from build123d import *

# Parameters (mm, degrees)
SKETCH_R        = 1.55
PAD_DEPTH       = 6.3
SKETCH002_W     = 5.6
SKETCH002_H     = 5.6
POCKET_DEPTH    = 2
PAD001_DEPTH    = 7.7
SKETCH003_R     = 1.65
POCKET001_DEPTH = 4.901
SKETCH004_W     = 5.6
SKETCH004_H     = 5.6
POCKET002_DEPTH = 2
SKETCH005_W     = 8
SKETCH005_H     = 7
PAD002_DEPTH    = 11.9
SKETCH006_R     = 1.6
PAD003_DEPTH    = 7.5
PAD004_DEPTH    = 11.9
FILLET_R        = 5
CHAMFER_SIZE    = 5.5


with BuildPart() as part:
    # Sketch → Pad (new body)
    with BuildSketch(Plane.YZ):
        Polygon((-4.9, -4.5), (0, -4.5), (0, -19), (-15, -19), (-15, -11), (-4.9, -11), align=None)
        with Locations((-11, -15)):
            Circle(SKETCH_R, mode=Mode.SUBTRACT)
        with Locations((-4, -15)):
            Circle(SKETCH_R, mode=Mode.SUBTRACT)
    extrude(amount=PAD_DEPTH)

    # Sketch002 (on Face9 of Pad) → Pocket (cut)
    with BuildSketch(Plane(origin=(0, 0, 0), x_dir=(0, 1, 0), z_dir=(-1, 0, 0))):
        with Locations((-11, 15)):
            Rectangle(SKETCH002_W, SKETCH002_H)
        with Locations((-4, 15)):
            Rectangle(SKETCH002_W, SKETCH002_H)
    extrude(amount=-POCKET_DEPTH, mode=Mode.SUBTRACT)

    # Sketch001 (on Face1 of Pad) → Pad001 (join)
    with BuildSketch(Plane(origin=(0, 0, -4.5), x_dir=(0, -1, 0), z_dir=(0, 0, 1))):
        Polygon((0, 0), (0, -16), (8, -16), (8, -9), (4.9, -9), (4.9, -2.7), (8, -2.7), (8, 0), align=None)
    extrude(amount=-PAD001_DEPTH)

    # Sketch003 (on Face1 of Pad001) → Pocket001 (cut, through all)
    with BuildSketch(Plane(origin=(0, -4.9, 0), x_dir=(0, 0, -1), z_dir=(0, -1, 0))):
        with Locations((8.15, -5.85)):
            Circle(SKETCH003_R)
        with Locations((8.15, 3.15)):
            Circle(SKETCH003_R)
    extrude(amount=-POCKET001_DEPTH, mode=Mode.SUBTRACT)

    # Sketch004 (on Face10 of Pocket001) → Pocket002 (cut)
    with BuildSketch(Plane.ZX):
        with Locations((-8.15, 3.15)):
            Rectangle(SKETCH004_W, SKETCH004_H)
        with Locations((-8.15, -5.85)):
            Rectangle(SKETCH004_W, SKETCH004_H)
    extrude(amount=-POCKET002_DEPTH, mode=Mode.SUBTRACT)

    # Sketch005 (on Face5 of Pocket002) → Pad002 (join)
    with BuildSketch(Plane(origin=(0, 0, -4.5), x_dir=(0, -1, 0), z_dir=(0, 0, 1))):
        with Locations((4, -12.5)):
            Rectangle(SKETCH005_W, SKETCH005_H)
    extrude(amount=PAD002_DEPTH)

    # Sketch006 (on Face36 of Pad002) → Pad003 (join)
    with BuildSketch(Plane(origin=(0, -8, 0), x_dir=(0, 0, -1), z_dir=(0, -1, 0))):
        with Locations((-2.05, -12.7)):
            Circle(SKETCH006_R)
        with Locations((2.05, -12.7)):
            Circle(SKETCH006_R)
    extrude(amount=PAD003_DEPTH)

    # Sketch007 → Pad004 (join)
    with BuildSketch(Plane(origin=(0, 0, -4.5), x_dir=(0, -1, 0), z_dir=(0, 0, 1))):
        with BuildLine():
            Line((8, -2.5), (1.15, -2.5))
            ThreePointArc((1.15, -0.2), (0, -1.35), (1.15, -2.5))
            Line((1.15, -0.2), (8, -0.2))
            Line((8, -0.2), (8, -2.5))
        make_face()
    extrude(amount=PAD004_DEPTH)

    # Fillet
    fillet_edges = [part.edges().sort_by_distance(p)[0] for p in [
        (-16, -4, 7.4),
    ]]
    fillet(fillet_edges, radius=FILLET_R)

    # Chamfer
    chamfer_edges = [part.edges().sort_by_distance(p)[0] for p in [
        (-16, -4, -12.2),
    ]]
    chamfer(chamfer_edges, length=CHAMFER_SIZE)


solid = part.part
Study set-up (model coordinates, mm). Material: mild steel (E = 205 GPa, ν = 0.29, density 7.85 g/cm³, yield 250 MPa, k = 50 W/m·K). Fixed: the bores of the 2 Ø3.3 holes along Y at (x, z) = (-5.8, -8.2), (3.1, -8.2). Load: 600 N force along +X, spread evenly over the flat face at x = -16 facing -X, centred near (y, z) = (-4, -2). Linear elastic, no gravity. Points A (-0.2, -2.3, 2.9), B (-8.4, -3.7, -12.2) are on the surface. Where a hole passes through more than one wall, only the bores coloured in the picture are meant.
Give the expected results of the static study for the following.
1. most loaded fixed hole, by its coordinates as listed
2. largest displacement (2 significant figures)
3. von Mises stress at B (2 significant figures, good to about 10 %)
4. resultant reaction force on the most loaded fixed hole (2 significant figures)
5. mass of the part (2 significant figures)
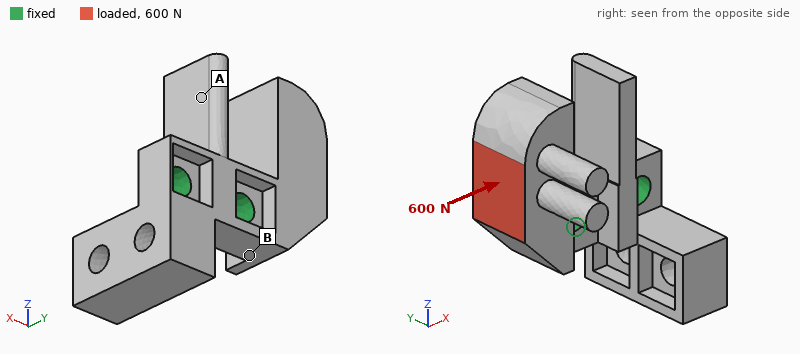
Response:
(-5.8, -8.2)
18 µm
49 MPa
620 N
18 g
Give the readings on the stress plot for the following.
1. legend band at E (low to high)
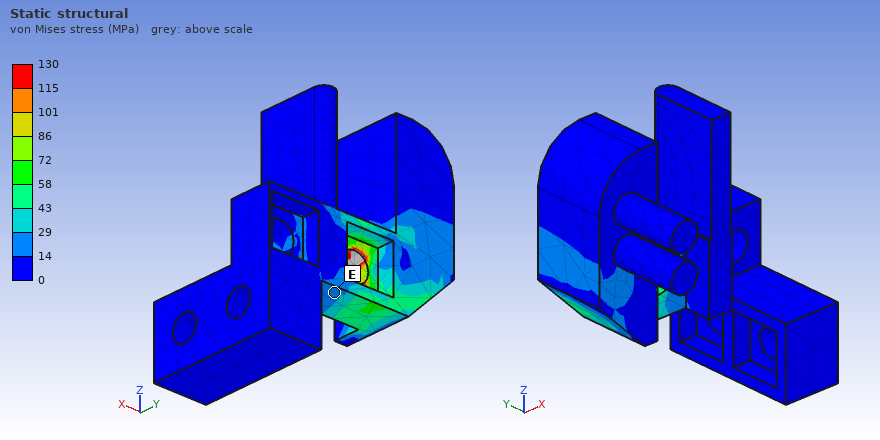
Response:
14 to 29 MPa
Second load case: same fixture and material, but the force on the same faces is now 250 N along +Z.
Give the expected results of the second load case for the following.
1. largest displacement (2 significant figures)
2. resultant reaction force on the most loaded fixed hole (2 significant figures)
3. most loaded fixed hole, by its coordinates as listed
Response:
9.3 µm
350 N
(-5.8, -8.2)
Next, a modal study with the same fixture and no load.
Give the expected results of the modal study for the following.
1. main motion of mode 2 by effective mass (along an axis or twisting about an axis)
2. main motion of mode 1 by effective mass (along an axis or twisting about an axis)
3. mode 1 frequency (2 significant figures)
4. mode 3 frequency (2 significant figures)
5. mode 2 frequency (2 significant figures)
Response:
along X
along Y
7700 Hz
11 kHz
10 kHz
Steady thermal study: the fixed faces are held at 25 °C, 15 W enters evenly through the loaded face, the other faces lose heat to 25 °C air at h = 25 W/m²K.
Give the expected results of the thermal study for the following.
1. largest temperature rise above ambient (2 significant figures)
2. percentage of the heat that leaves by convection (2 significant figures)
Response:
76 K
6.9 %
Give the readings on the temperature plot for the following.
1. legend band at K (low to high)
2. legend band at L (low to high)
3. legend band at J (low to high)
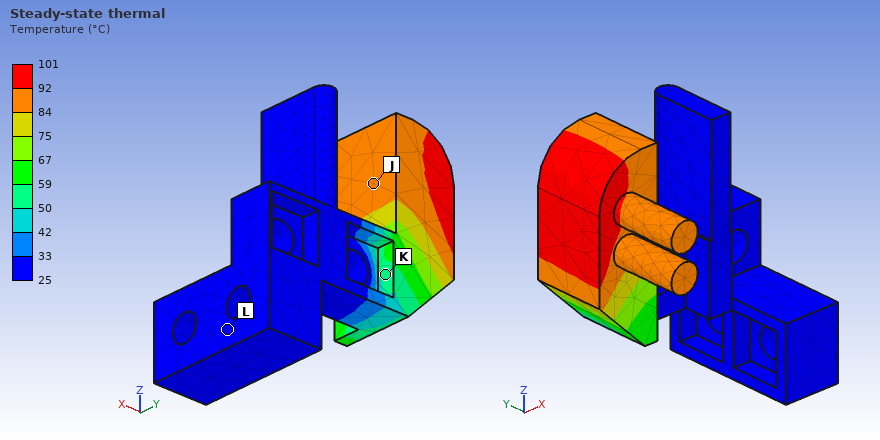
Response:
50 to 59 °C
25 to 33 °C
84 to 92 °C
